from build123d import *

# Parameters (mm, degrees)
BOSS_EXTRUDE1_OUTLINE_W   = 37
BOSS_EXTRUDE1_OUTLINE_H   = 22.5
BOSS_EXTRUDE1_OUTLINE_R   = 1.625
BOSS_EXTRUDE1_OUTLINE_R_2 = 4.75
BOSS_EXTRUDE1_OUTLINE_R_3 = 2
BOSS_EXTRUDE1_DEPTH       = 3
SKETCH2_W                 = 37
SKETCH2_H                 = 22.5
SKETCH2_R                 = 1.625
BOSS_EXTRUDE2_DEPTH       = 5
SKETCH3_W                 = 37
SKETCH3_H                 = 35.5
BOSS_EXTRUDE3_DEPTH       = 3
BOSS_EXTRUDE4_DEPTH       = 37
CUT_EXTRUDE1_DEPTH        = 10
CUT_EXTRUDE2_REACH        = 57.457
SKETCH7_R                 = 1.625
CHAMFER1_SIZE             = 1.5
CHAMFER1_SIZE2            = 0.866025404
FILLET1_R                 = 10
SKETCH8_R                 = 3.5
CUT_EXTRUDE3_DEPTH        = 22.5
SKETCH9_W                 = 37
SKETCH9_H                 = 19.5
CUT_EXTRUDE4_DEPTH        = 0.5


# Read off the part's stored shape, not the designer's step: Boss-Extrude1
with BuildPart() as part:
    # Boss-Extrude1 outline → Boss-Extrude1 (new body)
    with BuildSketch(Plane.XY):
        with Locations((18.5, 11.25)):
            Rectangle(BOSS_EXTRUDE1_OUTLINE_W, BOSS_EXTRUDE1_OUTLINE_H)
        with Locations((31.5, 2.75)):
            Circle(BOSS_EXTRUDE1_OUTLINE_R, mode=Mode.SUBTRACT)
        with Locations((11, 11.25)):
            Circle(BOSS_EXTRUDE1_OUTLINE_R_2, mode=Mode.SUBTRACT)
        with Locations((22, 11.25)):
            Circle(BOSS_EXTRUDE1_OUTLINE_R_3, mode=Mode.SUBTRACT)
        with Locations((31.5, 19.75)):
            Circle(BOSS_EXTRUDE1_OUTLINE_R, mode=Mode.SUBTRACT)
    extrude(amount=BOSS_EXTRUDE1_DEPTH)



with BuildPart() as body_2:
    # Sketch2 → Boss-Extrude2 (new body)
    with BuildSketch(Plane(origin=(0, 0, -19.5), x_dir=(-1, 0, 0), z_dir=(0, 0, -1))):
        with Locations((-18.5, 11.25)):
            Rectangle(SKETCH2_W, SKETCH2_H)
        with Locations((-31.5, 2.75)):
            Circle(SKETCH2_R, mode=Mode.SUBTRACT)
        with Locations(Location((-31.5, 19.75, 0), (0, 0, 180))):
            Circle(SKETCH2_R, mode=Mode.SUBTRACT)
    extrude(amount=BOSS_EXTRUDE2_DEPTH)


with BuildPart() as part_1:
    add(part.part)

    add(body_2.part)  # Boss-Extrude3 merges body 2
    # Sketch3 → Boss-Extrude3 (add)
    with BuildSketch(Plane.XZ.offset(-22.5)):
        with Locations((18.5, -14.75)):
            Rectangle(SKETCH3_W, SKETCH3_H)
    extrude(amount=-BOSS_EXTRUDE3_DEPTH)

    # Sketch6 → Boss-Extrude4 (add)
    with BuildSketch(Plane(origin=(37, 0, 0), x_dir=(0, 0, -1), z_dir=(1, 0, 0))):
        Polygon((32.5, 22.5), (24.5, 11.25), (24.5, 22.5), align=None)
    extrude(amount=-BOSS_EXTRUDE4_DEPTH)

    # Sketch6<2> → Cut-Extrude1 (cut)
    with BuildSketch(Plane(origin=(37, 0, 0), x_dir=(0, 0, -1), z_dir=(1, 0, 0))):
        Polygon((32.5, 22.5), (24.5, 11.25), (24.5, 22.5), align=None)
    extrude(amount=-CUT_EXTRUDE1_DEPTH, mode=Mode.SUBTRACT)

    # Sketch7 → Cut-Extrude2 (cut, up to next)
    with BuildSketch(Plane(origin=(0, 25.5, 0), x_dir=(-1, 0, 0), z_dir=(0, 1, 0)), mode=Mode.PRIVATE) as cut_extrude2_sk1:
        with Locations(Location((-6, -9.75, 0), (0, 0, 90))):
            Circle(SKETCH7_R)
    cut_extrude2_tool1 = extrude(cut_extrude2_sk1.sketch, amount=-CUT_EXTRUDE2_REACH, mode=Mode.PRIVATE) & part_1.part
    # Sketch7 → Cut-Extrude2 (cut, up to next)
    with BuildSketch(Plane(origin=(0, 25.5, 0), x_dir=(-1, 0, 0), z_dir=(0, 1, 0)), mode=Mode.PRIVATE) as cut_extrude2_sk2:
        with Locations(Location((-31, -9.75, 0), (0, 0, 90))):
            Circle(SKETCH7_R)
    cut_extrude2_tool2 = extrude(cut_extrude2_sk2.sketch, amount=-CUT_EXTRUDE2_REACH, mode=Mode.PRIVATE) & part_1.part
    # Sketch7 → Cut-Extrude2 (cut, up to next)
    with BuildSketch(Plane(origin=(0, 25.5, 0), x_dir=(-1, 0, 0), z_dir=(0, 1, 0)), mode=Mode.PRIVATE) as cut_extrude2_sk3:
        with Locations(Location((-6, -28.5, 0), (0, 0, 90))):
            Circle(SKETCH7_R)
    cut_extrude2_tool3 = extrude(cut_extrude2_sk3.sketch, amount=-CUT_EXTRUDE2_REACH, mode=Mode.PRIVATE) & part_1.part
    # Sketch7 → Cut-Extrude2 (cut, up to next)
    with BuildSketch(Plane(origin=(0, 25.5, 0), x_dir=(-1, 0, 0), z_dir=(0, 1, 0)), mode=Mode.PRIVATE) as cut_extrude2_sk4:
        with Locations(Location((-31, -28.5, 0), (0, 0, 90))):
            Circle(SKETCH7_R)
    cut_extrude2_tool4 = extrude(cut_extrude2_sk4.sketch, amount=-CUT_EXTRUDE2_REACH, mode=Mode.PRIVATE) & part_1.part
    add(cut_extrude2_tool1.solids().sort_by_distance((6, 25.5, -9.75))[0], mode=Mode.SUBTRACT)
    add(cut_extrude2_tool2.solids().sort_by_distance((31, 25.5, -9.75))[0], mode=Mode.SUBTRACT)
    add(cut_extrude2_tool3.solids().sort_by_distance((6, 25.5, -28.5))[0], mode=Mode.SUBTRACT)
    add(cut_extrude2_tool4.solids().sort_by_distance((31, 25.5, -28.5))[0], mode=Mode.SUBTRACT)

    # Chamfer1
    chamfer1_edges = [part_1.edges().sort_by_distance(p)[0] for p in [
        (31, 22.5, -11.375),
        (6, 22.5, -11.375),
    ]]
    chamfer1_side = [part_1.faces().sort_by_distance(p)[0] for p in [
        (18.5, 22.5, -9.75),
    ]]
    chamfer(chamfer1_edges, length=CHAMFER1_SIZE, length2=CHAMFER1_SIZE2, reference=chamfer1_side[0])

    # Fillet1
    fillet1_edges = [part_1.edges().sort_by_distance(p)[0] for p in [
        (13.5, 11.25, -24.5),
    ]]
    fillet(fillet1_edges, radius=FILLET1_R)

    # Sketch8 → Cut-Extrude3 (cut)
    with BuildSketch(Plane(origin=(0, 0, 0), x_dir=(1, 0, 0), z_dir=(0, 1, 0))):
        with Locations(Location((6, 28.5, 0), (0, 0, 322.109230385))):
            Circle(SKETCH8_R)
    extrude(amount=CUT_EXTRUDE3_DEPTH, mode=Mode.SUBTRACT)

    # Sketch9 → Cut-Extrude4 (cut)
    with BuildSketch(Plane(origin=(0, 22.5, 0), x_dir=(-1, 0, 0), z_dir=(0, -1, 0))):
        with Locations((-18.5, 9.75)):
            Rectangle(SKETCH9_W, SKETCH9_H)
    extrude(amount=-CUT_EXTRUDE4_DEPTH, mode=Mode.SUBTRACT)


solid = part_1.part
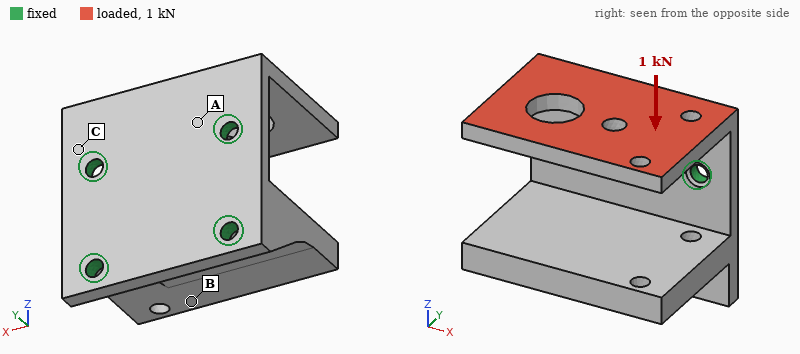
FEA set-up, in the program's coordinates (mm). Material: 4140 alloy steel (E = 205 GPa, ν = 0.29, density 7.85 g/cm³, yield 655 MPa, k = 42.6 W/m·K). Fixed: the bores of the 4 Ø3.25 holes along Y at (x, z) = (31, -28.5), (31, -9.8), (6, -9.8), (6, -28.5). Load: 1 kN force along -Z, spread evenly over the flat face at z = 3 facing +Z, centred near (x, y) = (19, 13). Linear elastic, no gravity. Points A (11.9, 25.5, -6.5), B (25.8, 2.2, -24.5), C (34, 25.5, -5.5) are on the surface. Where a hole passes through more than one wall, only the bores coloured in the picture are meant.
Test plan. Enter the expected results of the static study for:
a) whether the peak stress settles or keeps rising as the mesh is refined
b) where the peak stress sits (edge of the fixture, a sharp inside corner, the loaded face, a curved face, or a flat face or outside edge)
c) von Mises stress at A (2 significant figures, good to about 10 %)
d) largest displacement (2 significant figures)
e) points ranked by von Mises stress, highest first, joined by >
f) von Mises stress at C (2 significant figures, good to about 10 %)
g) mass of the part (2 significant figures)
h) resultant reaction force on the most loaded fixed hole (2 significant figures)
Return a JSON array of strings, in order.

["keeps rising", "edge of the fixture", "220 MPa", "0.41 mm", "C > A > B", "290 MPa", "85 g", "400 N"]
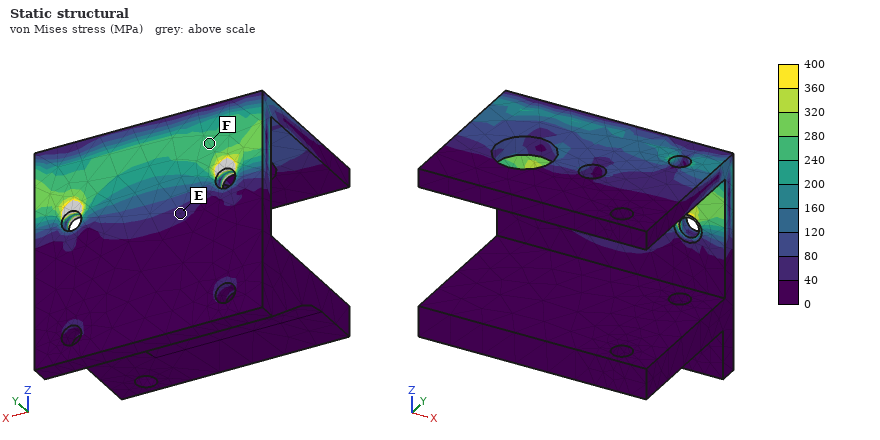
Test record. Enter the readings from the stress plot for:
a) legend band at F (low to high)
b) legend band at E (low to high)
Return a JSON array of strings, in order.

["240 to 280 MPa", "40 to 80 MPa"]
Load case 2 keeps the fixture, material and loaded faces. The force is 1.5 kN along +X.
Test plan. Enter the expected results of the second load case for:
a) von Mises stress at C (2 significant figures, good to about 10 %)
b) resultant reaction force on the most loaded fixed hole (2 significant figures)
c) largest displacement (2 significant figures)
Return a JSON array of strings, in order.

["140 MPa", "1.2 kN", "85 µm"]
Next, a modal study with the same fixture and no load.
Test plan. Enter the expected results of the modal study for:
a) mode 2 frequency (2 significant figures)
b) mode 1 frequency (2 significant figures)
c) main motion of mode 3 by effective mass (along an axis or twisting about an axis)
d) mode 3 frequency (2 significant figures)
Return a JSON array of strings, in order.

["4500 Hz", "2100 Hz", "along Z", "6600 Hz"]
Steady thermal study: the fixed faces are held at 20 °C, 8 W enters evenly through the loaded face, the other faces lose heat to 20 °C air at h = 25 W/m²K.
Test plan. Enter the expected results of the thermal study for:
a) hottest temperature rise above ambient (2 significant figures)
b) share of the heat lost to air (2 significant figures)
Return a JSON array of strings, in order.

["41 K", "18 %"]
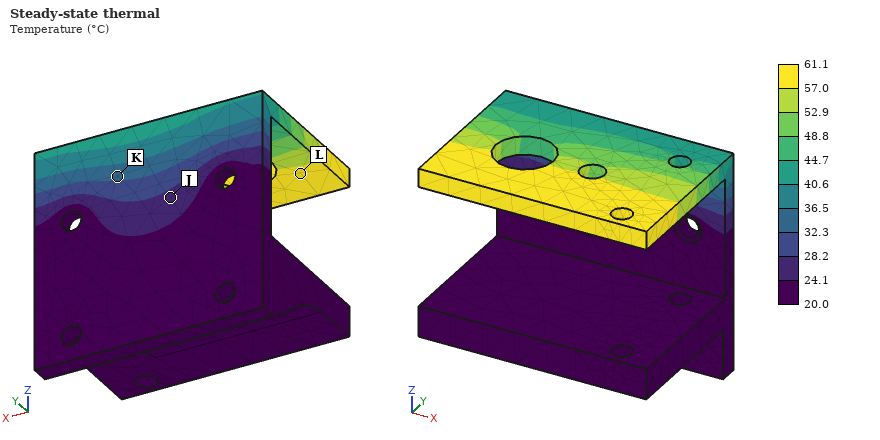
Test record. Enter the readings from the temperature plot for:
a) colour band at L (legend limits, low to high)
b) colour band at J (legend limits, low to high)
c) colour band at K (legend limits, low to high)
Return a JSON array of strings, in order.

["57.0 to 61.1 °C", "24.1 to 28.2 °C", "32.3 to 36.5 °C"]
